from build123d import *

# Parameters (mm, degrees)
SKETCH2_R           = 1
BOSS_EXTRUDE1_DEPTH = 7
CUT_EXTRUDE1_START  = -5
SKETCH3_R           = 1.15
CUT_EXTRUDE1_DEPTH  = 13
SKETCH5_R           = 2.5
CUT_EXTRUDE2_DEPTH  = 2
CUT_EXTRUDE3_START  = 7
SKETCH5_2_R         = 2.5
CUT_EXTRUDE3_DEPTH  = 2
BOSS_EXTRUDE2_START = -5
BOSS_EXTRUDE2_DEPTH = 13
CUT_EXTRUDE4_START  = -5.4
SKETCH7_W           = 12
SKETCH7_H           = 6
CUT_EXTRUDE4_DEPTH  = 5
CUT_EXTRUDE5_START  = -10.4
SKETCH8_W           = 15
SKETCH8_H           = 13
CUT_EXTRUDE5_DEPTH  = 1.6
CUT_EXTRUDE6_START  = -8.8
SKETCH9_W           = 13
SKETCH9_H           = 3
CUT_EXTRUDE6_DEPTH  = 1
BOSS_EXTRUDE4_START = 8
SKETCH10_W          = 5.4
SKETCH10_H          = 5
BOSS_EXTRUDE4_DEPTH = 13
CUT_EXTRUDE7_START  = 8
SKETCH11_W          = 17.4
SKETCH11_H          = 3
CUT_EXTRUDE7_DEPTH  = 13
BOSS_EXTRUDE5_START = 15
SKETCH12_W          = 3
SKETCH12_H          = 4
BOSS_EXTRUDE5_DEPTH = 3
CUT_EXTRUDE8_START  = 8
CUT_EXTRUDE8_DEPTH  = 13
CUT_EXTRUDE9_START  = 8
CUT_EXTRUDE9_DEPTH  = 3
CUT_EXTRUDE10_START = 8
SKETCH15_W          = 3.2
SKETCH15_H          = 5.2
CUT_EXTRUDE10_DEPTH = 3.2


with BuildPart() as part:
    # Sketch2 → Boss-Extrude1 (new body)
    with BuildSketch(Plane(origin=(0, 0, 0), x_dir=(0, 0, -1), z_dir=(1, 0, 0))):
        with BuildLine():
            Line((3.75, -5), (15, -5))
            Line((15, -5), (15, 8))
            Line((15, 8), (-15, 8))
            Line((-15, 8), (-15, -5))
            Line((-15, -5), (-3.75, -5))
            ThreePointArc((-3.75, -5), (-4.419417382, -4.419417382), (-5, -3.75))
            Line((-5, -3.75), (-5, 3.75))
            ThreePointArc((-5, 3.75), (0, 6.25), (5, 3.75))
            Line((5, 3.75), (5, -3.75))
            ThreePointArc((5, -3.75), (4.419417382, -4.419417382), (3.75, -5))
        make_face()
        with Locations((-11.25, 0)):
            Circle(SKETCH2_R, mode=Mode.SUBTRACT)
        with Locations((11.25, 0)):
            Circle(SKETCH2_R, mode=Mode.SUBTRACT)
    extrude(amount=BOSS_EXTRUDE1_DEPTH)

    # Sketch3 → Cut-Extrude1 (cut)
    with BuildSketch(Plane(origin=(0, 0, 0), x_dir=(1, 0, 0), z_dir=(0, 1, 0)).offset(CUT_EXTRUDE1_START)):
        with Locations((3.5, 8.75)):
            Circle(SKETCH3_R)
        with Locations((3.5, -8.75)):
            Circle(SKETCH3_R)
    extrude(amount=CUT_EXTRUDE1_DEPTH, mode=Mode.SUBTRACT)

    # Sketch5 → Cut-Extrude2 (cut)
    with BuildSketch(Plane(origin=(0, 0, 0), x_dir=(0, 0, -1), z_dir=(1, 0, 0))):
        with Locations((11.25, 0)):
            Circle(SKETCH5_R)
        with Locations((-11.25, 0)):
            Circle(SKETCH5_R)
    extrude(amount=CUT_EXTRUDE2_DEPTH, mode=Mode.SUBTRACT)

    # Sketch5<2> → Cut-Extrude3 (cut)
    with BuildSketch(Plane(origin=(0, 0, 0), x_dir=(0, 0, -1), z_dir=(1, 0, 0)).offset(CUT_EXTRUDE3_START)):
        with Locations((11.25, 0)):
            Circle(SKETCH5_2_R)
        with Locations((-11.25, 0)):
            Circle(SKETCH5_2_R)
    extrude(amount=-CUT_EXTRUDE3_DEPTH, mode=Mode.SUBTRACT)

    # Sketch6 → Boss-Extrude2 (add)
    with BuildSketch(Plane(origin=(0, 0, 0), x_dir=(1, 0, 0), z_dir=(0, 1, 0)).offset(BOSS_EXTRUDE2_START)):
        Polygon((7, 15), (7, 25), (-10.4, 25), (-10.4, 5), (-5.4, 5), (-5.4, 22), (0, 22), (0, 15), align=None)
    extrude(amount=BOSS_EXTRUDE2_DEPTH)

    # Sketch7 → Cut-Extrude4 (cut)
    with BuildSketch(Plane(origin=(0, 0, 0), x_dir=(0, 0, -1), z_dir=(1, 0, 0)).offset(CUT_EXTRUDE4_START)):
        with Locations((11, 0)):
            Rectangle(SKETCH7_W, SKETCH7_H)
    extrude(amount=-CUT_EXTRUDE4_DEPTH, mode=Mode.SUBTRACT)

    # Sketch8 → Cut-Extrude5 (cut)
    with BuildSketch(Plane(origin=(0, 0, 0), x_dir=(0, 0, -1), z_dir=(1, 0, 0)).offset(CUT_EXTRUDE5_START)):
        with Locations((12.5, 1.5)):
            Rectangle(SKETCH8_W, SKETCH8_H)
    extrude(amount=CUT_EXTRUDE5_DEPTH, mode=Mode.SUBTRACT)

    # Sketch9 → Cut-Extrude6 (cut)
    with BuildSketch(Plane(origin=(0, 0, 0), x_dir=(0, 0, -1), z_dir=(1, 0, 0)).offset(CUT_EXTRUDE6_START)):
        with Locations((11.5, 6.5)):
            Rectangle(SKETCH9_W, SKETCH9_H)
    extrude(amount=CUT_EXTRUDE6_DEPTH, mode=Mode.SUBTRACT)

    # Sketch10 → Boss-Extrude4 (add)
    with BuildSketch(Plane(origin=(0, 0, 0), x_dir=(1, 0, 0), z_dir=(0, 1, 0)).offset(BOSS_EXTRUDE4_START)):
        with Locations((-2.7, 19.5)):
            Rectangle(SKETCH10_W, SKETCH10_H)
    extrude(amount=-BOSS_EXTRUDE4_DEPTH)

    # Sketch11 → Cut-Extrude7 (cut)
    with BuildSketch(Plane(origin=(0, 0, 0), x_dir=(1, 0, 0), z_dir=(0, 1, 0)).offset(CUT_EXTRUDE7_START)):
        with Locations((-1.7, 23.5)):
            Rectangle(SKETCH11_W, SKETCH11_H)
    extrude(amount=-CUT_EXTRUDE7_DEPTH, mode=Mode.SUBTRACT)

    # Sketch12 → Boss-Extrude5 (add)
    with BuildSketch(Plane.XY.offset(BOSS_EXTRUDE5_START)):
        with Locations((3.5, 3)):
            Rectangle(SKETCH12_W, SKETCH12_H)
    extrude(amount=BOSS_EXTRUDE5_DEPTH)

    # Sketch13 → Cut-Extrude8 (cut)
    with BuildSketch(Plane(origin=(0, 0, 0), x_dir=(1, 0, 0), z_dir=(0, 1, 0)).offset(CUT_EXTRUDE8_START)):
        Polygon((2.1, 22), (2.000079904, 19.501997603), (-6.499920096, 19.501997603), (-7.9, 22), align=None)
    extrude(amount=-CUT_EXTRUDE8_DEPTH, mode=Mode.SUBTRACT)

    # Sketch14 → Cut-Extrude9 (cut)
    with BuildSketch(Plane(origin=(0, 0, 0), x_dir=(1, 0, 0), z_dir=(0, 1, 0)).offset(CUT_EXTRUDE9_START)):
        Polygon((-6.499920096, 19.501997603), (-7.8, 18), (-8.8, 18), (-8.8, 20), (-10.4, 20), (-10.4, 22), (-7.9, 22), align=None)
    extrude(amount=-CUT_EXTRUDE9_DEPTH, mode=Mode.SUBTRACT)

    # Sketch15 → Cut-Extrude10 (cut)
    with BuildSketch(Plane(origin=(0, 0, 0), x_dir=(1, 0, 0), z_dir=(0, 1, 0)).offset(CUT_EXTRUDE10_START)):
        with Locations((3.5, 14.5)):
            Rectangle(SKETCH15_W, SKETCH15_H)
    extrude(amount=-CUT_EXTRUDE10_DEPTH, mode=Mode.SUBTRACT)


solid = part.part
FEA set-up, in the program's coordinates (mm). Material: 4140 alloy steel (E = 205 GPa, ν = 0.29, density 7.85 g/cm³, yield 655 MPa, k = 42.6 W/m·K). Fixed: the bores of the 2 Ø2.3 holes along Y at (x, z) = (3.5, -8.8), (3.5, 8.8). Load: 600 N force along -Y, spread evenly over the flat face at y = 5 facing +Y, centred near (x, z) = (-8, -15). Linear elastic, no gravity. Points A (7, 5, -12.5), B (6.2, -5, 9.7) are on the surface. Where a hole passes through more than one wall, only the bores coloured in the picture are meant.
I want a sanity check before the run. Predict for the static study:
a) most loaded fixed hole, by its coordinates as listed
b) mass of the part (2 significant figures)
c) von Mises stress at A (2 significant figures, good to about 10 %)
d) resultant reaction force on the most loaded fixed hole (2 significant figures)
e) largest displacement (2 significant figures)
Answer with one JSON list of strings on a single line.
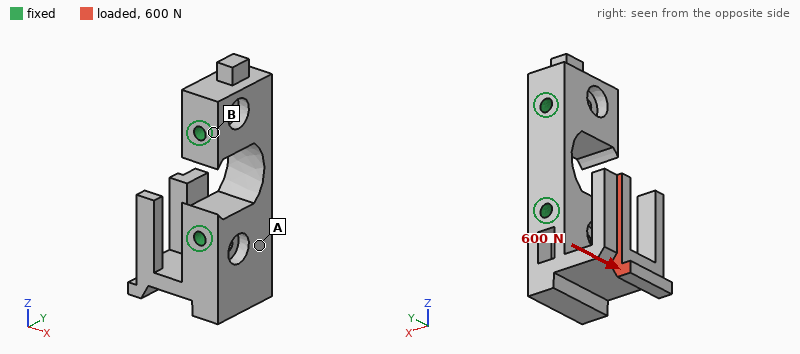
["(3.5, -8.8)", "23 g", "84 MPa", "600 N", "83 µm"]
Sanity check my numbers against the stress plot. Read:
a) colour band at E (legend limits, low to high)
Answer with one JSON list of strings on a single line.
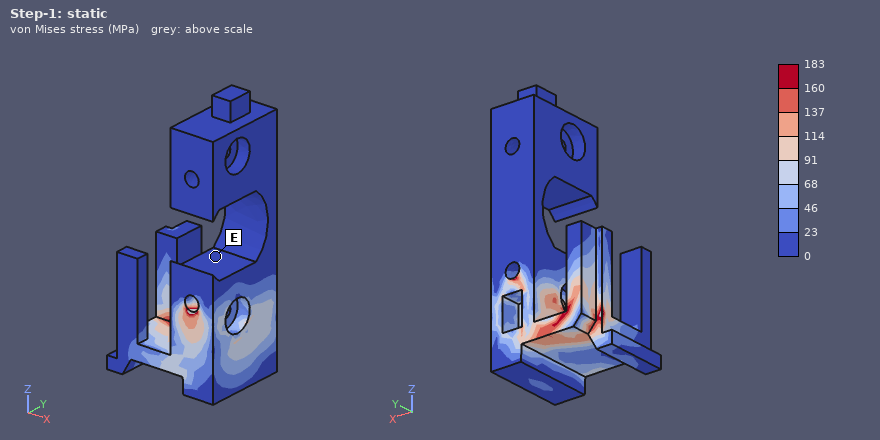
["0 to 23 MPa"]
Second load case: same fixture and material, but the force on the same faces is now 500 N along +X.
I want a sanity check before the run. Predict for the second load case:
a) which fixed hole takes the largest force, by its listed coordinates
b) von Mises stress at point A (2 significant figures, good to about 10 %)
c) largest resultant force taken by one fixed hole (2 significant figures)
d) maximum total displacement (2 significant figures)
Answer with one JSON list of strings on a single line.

["(3.5, -8.8)", "40 MPa", "530 N", "90 µm"]
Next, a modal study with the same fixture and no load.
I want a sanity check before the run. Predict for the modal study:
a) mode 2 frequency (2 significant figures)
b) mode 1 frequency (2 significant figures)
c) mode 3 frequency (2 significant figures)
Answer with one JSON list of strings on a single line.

["8100 Hz", "6500 Hz", "11 kHz"]
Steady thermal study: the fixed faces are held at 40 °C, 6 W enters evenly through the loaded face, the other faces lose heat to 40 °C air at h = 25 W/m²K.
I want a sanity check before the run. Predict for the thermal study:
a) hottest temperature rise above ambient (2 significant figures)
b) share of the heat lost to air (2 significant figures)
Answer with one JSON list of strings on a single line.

["88 K", "17 %"]
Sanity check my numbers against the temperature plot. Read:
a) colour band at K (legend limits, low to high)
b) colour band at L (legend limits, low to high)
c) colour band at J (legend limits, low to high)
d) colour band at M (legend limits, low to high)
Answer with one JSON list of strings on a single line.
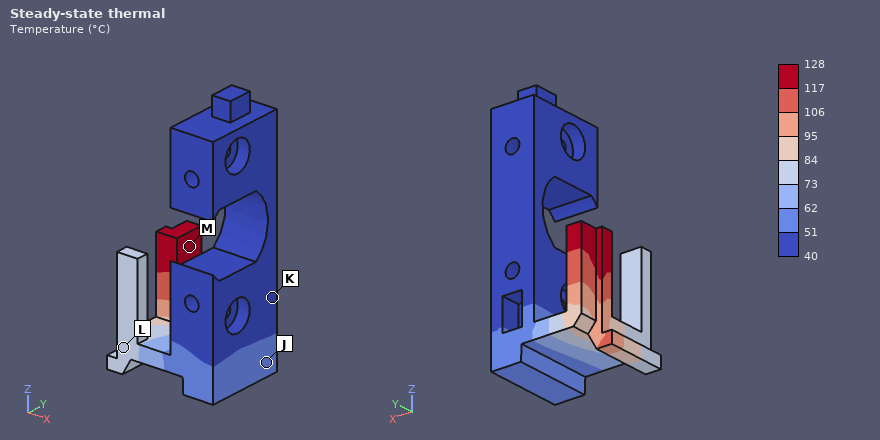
["40 to 51 °C", "73 to 84 °C", "51 to 62 °C", "117 to 128 °C"]
